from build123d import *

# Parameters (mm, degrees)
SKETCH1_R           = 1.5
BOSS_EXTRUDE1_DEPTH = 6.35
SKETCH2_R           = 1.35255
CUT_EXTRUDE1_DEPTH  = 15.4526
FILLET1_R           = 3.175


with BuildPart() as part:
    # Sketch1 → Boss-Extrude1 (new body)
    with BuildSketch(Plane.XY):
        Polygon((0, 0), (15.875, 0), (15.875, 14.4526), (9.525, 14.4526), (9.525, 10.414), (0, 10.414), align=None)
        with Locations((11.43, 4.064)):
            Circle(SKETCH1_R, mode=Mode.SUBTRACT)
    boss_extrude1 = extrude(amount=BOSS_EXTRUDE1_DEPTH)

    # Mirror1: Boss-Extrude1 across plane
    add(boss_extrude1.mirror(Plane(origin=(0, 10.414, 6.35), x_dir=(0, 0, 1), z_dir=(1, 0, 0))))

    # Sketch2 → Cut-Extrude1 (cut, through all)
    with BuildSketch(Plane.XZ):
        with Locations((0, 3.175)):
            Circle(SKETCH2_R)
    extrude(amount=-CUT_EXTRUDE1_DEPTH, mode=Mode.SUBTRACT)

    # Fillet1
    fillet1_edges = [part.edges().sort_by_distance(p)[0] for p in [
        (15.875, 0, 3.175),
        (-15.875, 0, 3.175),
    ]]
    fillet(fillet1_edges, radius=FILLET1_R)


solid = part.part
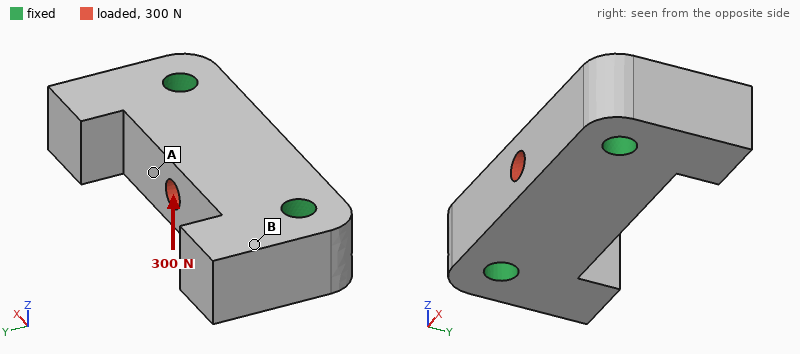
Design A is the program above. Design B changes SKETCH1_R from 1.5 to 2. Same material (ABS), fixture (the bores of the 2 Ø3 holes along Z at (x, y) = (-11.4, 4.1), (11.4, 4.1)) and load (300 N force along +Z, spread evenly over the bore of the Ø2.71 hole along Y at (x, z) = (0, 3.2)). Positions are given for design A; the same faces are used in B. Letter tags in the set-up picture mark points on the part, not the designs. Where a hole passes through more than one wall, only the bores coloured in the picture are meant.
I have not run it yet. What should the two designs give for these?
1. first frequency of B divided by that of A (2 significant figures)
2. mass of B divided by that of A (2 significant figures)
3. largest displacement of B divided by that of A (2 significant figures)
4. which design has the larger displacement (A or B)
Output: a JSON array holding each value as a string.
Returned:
["1.2", "0.97", "0.87", "A"]
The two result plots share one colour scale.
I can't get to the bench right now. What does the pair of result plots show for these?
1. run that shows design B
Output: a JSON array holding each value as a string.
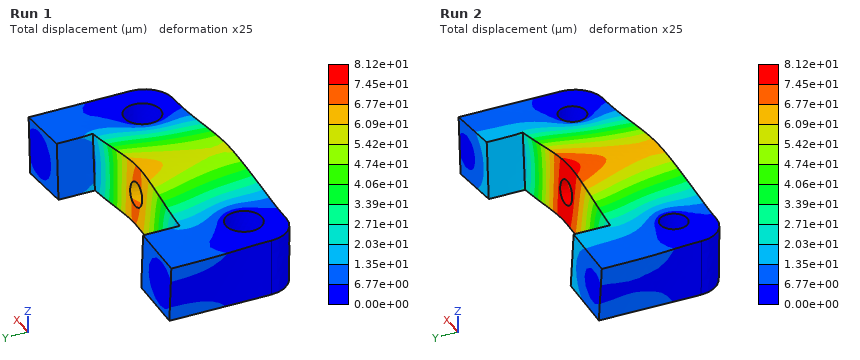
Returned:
["Run 1"]
